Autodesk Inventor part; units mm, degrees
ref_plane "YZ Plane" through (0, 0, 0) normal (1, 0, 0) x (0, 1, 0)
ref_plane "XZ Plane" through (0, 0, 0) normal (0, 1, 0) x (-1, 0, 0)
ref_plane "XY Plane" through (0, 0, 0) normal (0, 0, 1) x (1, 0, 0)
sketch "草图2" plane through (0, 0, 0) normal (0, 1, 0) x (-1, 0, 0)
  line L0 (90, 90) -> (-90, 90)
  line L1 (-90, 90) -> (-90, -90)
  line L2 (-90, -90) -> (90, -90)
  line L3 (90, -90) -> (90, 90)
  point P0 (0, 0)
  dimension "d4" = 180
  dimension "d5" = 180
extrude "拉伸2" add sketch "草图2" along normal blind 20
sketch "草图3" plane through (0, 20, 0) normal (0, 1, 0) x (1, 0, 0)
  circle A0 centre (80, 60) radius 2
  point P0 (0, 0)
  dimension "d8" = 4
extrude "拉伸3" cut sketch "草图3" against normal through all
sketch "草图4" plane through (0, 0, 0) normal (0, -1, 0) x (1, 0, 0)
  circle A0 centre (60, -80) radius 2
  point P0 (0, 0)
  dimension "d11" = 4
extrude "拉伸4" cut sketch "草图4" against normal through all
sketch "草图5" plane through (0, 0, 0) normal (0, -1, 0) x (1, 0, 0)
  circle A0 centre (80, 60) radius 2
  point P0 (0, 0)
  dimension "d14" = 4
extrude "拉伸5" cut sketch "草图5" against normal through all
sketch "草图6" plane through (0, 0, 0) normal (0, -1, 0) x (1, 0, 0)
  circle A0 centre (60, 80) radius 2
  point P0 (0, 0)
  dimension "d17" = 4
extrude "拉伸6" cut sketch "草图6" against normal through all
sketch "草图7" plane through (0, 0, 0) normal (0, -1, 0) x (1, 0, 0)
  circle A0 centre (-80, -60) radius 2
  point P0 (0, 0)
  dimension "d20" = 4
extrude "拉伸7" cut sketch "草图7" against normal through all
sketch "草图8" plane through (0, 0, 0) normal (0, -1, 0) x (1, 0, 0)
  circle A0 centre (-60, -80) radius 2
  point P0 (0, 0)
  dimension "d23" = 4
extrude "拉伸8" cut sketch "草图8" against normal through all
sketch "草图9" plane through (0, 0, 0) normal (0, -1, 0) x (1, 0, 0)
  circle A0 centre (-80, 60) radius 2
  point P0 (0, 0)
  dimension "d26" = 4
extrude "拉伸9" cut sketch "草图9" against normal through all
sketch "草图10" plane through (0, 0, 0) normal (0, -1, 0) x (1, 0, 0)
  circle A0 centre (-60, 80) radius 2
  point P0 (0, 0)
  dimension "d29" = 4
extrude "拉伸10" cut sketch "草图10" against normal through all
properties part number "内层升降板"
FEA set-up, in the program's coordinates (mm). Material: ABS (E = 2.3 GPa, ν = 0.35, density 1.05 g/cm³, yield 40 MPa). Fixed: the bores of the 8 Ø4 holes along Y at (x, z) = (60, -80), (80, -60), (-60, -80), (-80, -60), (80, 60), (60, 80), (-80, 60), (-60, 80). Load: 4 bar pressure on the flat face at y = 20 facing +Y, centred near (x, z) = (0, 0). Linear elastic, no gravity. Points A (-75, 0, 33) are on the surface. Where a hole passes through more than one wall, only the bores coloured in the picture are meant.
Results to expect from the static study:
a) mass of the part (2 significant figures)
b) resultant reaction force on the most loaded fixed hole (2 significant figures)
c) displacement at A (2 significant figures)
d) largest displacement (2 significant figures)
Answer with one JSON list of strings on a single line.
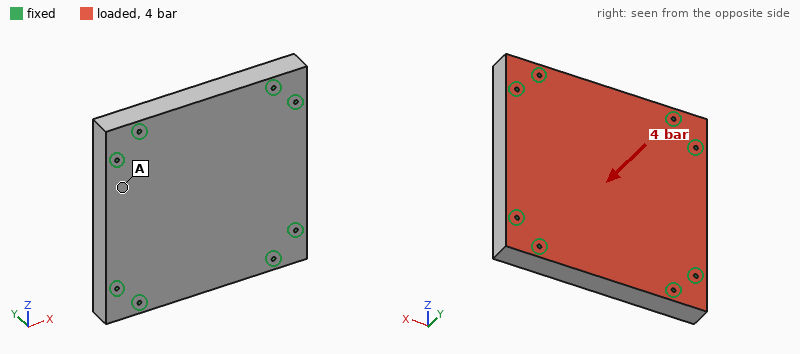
["680 g", "1.6 kN", "0.28 mm", "0.83 mm"]
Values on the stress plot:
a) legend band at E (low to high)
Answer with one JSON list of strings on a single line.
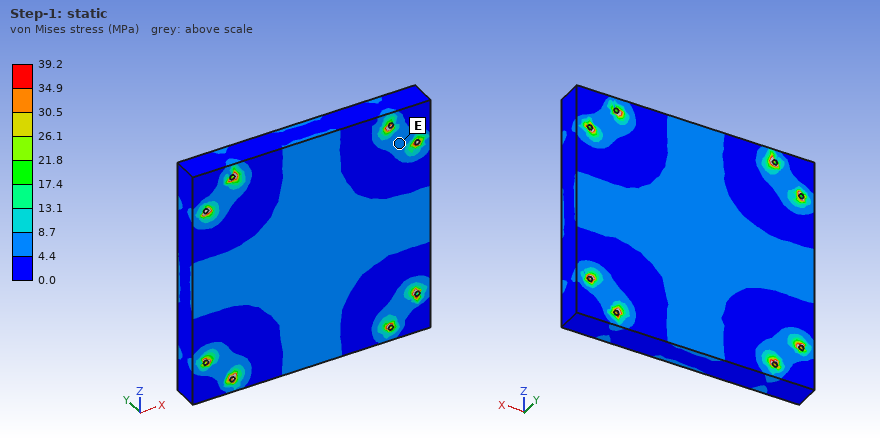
["4.4 to 8.7 MPa"]
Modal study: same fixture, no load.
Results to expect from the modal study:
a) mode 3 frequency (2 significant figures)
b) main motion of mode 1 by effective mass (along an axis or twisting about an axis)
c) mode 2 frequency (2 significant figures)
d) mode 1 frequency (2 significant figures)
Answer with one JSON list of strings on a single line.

["1600 Hz", "along Y", "1600 Hz", "920 Hz"]
